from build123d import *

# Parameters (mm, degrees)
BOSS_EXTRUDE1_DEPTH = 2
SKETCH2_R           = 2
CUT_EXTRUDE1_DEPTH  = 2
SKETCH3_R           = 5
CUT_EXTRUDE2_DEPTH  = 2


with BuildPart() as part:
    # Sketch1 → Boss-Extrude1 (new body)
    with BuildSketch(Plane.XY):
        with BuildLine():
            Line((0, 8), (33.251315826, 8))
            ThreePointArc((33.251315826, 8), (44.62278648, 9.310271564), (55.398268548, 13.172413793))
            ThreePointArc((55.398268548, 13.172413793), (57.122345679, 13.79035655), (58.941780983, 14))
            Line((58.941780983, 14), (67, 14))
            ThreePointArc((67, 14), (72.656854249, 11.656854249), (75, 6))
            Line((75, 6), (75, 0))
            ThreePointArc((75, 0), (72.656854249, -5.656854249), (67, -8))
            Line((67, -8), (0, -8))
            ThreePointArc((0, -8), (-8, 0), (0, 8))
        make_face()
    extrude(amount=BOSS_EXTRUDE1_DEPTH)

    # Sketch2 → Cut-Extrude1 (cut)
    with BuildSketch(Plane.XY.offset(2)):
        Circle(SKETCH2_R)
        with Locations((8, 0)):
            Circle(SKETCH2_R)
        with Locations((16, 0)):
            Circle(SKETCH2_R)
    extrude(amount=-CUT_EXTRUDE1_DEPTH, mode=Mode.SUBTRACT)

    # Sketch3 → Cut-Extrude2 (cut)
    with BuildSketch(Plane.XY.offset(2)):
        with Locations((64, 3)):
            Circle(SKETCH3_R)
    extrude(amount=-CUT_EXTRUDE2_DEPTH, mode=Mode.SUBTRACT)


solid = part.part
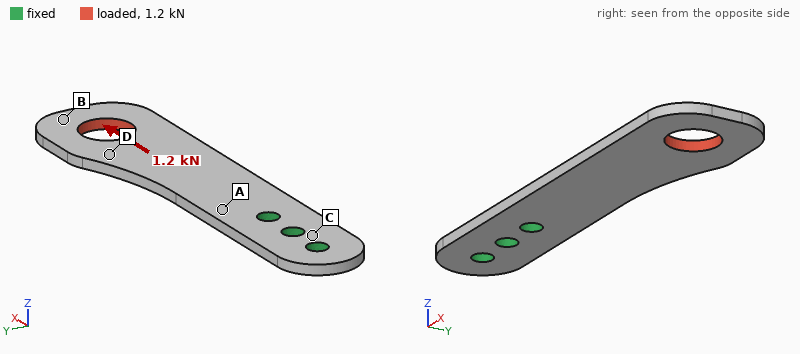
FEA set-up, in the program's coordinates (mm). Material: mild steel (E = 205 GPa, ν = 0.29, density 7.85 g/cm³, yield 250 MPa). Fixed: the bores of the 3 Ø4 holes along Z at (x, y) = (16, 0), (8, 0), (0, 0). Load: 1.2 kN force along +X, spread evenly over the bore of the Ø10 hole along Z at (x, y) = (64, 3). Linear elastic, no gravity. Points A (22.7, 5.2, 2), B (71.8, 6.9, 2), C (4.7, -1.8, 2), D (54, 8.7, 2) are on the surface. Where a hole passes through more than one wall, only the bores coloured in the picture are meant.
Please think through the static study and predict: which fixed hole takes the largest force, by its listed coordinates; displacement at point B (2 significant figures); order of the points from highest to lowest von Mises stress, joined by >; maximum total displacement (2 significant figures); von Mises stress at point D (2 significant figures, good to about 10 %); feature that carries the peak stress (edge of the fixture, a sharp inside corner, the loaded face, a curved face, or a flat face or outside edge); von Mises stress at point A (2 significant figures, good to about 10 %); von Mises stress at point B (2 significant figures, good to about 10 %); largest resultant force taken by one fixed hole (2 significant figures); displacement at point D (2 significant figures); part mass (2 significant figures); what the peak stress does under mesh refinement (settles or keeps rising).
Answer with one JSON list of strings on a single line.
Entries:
["(16, 0)", "44 µm", "A > D > B > C", "47 µm", "40 MPa", "edge of the fixture", "62 MPa", "22 MPa", "960 N", "28 µm", "21 g", "keeps rising"]
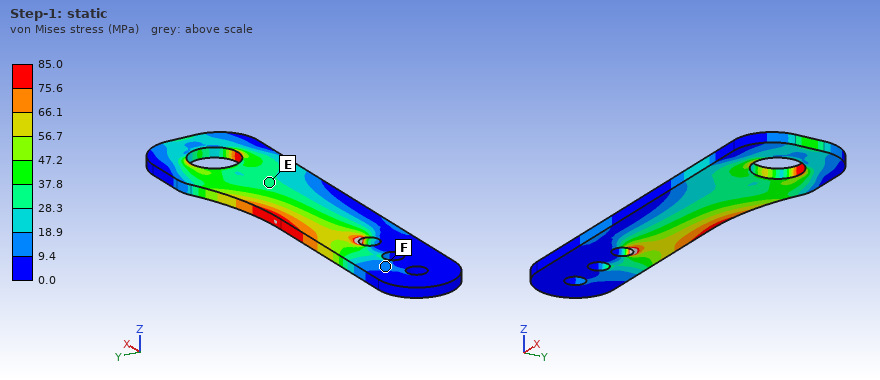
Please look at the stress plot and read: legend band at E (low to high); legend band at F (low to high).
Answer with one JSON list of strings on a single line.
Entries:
["28.3 to 37.8 MPa", "9.4 to 18.9 MPa"]
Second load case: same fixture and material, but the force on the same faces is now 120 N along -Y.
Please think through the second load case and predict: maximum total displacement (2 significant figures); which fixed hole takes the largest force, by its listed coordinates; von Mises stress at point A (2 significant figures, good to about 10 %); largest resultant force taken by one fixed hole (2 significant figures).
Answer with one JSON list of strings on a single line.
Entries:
["58 µm", "(16, 0)", "38 MPa", "420 N"]
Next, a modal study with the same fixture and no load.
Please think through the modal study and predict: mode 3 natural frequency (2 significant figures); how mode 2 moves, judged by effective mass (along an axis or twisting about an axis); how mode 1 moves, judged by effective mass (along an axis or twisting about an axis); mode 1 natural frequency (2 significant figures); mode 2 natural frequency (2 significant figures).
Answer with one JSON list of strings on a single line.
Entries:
["3000 Hz", "twisting about X", "along Z", "480 Hz", "2500 Hz"]
